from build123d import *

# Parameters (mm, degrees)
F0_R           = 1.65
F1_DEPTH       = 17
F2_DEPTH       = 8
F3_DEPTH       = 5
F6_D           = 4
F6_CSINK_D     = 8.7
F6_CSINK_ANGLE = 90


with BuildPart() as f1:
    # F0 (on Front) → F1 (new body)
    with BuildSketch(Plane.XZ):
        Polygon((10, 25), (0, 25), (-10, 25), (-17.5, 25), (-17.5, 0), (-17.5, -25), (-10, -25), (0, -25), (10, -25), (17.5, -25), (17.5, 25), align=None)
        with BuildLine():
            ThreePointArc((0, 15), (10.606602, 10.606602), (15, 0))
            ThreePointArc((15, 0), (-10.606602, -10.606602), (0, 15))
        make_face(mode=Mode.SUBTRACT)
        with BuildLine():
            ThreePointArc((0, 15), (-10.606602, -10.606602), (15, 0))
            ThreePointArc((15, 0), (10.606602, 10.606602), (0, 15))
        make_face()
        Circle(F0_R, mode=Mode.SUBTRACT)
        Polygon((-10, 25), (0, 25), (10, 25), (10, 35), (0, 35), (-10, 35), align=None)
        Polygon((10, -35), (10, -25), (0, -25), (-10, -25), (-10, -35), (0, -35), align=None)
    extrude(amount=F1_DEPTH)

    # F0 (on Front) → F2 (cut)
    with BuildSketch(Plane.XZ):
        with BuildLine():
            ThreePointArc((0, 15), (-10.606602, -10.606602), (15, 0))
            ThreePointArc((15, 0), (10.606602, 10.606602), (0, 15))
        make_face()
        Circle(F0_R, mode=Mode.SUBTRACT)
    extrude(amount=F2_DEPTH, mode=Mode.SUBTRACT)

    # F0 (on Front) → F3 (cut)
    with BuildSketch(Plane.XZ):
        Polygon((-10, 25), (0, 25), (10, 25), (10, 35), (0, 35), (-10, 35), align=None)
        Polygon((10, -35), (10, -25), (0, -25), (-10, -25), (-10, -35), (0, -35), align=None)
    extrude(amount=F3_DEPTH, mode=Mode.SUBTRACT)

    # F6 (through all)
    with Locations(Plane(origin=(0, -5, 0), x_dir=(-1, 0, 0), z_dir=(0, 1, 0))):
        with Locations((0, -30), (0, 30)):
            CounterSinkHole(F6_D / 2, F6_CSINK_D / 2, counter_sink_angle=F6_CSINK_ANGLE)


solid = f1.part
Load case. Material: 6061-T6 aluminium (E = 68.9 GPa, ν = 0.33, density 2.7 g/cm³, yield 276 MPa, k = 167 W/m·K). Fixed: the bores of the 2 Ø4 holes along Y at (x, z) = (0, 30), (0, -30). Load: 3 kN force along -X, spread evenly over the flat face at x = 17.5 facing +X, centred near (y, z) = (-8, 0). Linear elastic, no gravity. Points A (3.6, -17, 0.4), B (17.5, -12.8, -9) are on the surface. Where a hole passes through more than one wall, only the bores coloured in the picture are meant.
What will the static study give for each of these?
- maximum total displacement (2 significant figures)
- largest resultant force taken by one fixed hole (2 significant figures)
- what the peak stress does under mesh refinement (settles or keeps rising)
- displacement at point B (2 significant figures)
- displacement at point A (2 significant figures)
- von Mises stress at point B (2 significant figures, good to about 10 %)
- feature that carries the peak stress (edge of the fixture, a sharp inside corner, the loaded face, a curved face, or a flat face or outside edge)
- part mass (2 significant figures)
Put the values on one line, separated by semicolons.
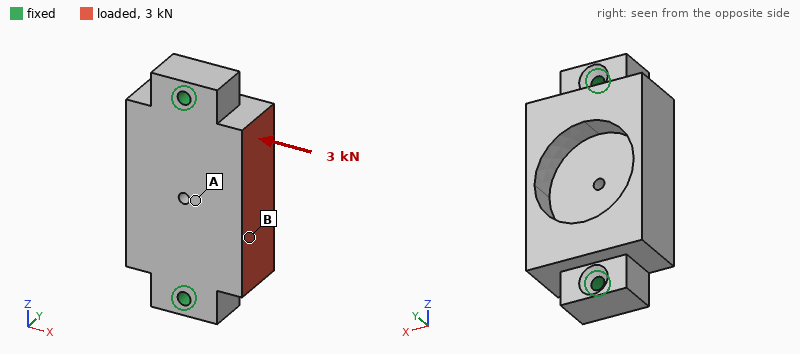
18 µm; 1.5 kN; keeps rising; 8.5 µm; 4.3 µm; 9.4 MPa; edge of the fixture; 77 g
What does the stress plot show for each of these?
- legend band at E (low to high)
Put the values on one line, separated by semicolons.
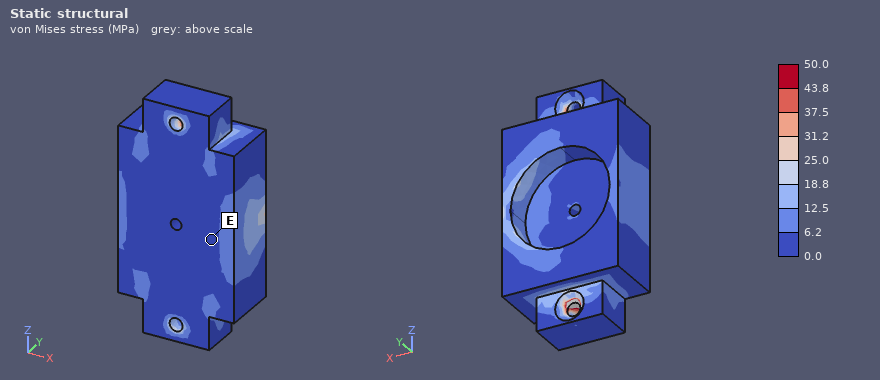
0.0 to 6.2 MPa
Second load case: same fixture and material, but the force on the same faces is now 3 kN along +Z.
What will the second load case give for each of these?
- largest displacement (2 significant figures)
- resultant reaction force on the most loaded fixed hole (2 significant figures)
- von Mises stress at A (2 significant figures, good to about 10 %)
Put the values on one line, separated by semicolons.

6.7 µm; 1.7 kN; 6.6 MPa
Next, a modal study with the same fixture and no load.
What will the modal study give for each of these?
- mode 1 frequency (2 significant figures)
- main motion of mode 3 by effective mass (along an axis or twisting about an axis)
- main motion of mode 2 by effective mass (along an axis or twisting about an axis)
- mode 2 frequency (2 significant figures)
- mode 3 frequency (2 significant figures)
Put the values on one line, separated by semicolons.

8900 Hz; along X; along Y; 9700 Hz; 16 kHz
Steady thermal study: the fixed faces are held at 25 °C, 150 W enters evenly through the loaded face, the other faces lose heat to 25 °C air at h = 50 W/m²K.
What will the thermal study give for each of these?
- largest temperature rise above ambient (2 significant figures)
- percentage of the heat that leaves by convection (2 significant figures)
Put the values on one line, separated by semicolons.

51 K; 5.0 %
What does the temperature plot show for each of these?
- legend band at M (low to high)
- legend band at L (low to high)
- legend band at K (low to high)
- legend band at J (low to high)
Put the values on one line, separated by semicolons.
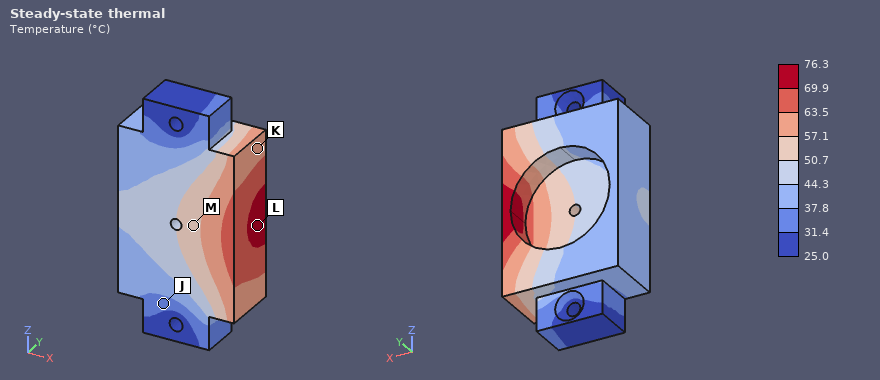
50.7 to 57.1 °C; 69.9 to 76.3 °C; 57.1 to 63.5 °C; 31.4 to 37.8 °C
